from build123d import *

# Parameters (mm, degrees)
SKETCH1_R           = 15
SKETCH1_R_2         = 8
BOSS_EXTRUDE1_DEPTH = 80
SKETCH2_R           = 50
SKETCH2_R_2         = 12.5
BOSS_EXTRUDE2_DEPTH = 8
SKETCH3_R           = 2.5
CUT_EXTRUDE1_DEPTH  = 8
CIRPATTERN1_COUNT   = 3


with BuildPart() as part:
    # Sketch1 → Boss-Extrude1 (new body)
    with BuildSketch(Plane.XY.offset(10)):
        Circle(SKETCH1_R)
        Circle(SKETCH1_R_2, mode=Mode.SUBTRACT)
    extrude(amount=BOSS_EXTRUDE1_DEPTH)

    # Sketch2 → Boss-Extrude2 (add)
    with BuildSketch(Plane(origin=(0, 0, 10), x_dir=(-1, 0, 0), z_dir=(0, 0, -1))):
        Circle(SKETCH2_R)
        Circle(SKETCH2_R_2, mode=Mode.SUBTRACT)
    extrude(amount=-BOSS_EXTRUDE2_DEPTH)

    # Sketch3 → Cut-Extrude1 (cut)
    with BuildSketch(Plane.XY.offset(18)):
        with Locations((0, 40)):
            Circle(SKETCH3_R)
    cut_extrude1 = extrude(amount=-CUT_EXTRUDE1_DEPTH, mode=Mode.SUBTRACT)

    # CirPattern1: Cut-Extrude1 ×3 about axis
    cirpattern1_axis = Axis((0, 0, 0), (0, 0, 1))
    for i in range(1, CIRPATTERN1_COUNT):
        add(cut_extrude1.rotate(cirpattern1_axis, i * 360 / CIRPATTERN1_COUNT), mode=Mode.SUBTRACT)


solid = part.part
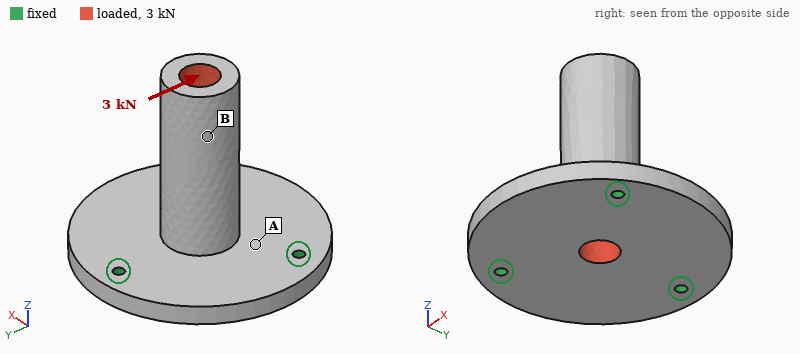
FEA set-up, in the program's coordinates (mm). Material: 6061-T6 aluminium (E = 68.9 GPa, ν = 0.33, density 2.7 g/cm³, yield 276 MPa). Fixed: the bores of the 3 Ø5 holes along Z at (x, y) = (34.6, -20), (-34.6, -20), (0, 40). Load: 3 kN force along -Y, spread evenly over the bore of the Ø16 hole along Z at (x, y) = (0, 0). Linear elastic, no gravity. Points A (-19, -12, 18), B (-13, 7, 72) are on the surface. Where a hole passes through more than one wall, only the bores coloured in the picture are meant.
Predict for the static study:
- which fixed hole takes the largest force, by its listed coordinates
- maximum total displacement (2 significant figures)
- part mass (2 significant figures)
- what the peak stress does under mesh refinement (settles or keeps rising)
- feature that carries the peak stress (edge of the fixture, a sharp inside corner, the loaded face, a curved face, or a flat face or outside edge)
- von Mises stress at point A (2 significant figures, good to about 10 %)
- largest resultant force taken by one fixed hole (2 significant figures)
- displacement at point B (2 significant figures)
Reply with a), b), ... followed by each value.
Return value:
a) (0, 40)
b) 0.23 mm
c) 260 g
d) keeps rising
e) edge of the fixture
f) 24 MPa
g) 2.2 kN
h) 0.17 mm
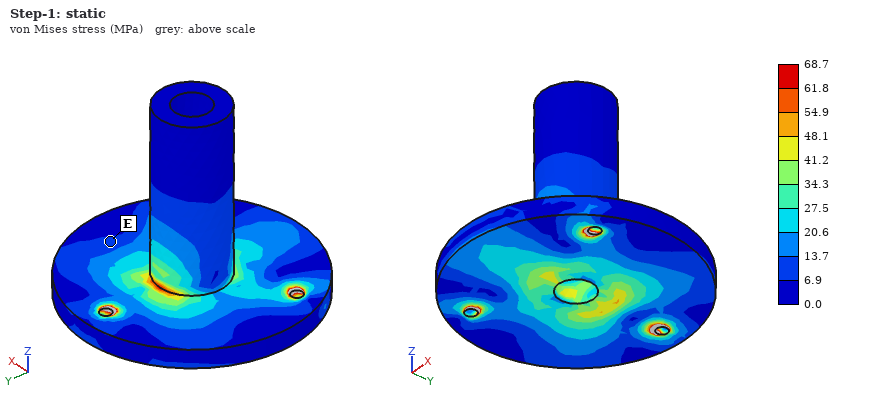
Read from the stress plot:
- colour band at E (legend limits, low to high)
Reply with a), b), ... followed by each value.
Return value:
a) 6.9 to 13.7 MPa
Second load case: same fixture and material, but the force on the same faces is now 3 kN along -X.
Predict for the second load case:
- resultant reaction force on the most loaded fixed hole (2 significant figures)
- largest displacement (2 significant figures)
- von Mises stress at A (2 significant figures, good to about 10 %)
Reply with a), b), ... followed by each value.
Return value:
a) 2.0 kN
b) 0.23 mm
c) 33 MPa
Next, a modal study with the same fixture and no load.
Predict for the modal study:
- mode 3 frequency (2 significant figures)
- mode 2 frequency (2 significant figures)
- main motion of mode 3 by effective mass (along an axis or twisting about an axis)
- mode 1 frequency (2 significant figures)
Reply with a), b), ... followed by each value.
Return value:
a) 4300 Hz
b) 2100 Hz
c) along Z
d) 2100 Hz
